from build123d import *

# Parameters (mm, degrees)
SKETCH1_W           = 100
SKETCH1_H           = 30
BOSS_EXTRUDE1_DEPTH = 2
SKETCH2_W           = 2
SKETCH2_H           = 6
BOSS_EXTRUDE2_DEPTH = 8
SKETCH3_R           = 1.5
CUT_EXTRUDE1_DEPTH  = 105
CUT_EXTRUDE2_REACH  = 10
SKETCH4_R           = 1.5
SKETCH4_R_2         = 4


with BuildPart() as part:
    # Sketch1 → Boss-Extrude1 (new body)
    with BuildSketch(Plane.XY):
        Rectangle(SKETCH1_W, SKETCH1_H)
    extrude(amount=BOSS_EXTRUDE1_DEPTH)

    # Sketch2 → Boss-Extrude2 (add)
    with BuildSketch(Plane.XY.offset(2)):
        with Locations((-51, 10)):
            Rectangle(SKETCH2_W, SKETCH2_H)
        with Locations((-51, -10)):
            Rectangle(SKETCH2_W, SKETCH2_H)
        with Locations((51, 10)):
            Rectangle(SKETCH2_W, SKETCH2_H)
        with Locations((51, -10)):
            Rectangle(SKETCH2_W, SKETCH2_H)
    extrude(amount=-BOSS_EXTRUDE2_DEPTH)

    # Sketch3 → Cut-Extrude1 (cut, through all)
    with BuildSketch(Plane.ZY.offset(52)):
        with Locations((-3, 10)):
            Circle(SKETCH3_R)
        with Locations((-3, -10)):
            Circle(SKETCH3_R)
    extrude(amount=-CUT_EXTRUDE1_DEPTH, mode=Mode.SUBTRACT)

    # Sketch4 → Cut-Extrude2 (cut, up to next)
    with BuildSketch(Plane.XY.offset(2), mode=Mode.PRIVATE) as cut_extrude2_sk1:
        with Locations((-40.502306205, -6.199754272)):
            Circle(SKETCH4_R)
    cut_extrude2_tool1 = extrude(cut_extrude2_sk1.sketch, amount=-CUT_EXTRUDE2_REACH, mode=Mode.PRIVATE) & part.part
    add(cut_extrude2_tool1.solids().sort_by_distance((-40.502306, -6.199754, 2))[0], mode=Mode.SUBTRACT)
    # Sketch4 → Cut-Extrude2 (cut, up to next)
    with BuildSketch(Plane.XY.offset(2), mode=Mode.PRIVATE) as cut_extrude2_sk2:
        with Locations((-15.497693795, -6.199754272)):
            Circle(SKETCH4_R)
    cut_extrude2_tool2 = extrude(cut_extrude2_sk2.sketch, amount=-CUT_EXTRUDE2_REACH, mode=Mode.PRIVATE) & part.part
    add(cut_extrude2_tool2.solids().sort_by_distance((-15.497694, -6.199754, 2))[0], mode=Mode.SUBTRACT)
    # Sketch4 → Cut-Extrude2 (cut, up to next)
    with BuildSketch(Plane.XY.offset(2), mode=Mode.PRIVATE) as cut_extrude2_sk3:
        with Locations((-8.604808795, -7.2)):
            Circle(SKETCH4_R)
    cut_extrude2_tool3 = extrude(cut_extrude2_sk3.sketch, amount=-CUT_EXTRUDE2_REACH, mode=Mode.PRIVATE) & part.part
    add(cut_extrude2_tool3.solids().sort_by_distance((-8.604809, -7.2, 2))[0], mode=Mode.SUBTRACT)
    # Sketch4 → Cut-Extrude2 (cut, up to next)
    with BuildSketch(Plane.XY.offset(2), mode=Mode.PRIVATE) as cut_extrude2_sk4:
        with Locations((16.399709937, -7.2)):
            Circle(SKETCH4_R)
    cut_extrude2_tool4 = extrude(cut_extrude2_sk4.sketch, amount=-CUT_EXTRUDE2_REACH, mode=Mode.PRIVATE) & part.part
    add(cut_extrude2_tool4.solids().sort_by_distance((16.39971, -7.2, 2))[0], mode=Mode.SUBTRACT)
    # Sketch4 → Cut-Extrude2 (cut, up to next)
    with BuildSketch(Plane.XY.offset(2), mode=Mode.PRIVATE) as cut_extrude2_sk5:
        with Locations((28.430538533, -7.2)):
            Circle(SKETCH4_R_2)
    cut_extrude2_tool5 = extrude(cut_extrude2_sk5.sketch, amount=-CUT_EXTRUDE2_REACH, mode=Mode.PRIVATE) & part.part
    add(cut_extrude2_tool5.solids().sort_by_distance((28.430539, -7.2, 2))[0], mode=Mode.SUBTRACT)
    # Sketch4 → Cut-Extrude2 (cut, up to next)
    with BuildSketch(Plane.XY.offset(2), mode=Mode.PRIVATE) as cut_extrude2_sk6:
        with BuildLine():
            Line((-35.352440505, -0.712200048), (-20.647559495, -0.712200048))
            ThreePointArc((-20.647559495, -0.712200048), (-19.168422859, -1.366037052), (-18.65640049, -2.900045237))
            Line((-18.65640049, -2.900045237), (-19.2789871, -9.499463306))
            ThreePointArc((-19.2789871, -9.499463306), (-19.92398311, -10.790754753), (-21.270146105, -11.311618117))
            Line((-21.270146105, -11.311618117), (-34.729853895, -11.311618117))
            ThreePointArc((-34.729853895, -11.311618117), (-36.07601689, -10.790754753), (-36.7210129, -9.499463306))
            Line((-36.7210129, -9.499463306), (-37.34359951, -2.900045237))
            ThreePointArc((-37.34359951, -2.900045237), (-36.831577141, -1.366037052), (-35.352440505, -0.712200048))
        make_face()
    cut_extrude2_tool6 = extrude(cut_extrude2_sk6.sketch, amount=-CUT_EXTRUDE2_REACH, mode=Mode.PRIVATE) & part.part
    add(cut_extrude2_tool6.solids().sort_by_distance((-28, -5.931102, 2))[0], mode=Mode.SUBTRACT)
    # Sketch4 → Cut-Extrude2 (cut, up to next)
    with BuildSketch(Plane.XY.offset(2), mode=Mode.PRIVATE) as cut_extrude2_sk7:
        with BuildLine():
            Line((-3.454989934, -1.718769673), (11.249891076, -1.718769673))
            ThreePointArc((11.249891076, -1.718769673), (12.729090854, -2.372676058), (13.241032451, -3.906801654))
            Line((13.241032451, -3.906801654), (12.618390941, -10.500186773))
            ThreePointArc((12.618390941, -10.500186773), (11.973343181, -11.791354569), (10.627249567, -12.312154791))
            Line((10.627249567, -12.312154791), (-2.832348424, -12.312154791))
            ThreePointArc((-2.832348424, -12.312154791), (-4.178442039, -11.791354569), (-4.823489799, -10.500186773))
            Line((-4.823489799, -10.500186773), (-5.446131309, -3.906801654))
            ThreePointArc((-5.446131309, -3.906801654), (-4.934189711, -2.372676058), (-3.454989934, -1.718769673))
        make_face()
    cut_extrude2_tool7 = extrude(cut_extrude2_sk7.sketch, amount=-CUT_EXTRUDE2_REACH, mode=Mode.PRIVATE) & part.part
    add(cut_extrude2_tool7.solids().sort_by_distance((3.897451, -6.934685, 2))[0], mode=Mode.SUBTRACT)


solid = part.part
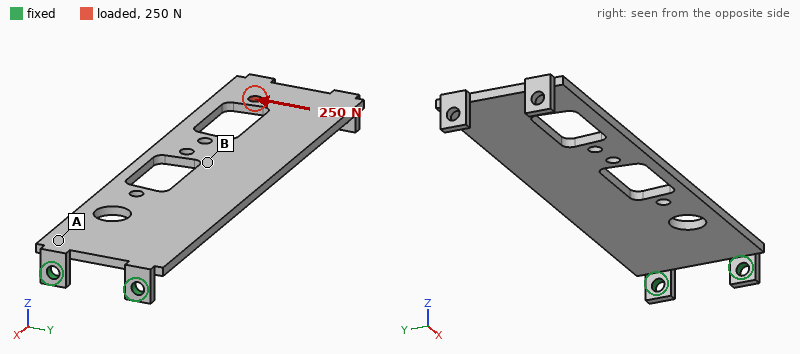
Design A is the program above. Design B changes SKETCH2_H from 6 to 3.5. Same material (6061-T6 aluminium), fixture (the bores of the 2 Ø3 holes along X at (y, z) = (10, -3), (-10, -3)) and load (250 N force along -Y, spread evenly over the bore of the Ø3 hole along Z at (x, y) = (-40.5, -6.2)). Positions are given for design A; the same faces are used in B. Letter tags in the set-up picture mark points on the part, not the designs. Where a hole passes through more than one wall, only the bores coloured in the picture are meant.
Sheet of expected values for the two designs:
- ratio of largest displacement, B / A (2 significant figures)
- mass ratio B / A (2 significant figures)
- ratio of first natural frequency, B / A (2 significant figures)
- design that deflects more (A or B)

1.2
0.97
0.95
B
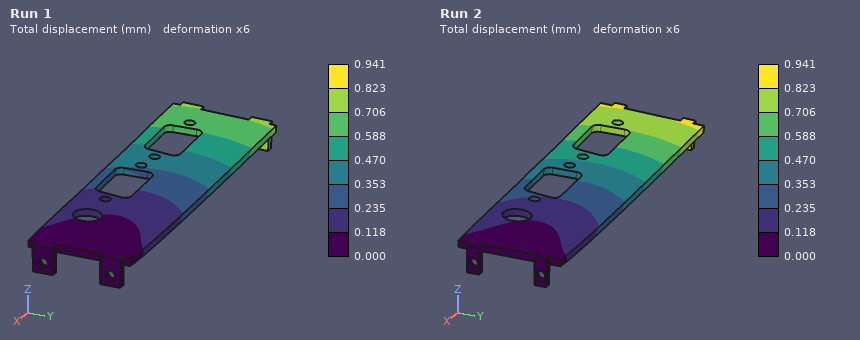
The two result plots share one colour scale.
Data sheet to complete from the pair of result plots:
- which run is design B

Run 2
